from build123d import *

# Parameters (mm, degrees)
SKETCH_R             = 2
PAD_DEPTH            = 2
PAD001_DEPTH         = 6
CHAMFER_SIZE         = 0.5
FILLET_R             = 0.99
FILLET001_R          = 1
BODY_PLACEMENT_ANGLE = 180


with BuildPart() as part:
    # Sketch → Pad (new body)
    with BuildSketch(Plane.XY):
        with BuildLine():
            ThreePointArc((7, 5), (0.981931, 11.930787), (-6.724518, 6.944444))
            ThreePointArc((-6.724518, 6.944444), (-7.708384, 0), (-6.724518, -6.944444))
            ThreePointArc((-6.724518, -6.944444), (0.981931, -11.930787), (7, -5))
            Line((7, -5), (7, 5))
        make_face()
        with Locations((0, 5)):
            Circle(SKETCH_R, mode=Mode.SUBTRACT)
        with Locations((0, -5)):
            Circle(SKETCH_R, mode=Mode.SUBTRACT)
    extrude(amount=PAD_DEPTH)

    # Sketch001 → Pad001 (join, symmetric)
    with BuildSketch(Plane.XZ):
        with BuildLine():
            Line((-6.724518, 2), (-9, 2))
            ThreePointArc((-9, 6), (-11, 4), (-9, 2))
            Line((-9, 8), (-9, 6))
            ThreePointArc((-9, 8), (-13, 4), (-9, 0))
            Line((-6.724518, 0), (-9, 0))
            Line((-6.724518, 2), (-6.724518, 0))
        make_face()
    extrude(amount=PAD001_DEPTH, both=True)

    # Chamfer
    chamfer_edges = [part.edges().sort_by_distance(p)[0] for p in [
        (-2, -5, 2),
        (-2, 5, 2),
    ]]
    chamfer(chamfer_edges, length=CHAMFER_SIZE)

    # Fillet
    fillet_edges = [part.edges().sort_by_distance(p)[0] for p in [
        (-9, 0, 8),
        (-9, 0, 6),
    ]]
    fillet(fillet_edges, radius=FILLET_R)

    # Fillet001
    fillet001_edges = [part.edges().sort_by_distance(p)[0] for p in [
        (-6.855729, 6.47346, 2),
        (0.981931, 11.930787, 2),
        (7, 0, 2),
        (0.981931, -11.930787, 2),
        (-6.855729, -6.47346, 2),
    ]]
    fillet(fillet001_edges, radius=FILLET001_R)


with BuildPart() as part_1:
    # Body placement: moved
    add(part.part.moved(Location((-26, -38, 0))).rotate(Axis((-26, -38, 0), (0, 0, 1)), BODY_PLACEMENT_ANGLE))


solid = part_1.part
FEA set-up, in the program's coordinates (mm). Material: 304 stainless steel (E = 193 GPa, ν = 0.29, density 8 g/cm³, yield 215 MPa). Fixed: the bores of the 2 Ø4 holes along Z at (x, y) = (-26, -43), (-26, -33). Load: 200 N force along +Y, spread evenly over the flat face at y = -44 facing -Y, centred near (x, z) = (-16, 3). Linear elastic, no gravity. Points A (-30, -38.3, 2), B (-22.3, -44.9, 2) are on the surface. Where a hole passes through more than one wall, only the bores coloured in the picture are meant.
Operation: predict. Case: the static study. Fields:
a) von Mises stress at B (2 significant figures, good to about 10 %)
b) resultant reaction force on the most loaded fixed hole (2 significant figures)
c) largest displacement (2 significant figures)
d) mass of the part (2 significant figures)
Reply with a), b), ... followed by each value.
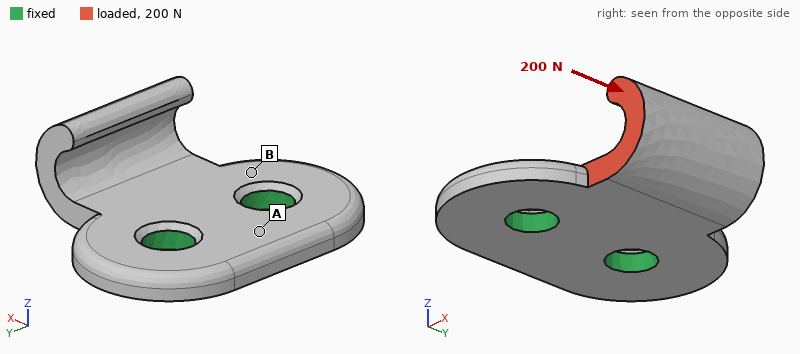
a) 11 MPa
b) 190 N
c) 11 µm
d) 6.3 g
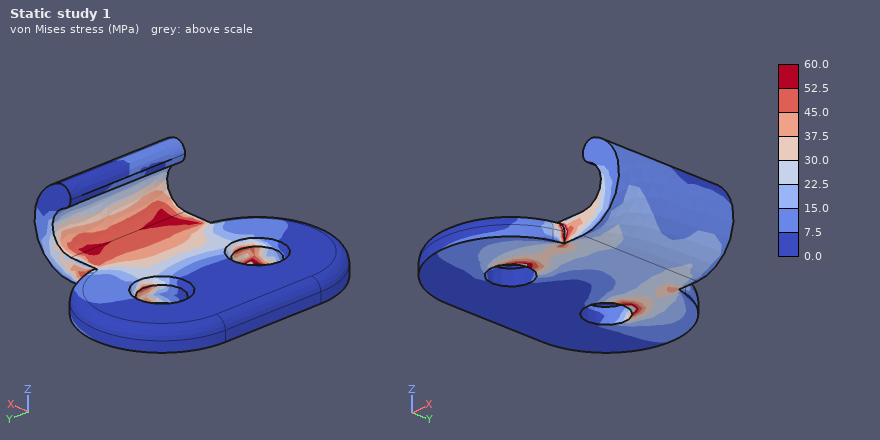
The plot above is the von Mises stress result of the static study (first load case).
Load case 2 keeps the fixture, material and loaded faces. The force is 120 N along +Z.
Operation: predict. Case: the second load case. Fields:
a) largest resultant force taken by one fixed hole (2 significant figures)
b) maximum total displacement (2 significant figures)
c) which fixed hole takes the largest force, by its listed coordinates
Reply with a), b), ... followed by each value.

a) 120 N
b) 35 µm
c) (-26, -43)
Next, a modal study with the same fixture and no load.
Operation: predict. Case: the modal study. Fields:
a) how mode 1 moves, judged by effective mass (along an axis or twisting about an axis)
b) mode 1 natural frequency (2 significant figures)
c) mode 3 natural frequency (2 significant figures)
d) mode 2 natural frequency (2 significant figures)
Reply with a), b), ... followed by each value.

a) along Z
b) 7700 Hz
c) 23 kHz
d) 15 kHz
